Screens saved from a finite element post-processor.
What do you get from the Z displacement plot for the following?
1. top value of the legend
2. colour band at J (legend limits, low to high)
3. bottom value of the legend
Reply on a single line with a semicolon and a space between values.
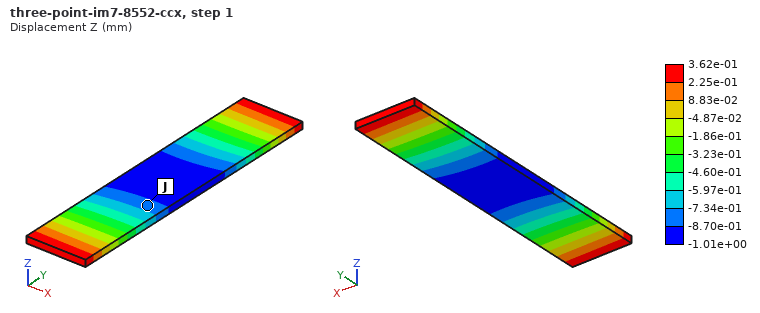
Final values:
3.62e-01 mm; -8.70e-01 to -7.34e-01 mm; -1.01e+00 mm
